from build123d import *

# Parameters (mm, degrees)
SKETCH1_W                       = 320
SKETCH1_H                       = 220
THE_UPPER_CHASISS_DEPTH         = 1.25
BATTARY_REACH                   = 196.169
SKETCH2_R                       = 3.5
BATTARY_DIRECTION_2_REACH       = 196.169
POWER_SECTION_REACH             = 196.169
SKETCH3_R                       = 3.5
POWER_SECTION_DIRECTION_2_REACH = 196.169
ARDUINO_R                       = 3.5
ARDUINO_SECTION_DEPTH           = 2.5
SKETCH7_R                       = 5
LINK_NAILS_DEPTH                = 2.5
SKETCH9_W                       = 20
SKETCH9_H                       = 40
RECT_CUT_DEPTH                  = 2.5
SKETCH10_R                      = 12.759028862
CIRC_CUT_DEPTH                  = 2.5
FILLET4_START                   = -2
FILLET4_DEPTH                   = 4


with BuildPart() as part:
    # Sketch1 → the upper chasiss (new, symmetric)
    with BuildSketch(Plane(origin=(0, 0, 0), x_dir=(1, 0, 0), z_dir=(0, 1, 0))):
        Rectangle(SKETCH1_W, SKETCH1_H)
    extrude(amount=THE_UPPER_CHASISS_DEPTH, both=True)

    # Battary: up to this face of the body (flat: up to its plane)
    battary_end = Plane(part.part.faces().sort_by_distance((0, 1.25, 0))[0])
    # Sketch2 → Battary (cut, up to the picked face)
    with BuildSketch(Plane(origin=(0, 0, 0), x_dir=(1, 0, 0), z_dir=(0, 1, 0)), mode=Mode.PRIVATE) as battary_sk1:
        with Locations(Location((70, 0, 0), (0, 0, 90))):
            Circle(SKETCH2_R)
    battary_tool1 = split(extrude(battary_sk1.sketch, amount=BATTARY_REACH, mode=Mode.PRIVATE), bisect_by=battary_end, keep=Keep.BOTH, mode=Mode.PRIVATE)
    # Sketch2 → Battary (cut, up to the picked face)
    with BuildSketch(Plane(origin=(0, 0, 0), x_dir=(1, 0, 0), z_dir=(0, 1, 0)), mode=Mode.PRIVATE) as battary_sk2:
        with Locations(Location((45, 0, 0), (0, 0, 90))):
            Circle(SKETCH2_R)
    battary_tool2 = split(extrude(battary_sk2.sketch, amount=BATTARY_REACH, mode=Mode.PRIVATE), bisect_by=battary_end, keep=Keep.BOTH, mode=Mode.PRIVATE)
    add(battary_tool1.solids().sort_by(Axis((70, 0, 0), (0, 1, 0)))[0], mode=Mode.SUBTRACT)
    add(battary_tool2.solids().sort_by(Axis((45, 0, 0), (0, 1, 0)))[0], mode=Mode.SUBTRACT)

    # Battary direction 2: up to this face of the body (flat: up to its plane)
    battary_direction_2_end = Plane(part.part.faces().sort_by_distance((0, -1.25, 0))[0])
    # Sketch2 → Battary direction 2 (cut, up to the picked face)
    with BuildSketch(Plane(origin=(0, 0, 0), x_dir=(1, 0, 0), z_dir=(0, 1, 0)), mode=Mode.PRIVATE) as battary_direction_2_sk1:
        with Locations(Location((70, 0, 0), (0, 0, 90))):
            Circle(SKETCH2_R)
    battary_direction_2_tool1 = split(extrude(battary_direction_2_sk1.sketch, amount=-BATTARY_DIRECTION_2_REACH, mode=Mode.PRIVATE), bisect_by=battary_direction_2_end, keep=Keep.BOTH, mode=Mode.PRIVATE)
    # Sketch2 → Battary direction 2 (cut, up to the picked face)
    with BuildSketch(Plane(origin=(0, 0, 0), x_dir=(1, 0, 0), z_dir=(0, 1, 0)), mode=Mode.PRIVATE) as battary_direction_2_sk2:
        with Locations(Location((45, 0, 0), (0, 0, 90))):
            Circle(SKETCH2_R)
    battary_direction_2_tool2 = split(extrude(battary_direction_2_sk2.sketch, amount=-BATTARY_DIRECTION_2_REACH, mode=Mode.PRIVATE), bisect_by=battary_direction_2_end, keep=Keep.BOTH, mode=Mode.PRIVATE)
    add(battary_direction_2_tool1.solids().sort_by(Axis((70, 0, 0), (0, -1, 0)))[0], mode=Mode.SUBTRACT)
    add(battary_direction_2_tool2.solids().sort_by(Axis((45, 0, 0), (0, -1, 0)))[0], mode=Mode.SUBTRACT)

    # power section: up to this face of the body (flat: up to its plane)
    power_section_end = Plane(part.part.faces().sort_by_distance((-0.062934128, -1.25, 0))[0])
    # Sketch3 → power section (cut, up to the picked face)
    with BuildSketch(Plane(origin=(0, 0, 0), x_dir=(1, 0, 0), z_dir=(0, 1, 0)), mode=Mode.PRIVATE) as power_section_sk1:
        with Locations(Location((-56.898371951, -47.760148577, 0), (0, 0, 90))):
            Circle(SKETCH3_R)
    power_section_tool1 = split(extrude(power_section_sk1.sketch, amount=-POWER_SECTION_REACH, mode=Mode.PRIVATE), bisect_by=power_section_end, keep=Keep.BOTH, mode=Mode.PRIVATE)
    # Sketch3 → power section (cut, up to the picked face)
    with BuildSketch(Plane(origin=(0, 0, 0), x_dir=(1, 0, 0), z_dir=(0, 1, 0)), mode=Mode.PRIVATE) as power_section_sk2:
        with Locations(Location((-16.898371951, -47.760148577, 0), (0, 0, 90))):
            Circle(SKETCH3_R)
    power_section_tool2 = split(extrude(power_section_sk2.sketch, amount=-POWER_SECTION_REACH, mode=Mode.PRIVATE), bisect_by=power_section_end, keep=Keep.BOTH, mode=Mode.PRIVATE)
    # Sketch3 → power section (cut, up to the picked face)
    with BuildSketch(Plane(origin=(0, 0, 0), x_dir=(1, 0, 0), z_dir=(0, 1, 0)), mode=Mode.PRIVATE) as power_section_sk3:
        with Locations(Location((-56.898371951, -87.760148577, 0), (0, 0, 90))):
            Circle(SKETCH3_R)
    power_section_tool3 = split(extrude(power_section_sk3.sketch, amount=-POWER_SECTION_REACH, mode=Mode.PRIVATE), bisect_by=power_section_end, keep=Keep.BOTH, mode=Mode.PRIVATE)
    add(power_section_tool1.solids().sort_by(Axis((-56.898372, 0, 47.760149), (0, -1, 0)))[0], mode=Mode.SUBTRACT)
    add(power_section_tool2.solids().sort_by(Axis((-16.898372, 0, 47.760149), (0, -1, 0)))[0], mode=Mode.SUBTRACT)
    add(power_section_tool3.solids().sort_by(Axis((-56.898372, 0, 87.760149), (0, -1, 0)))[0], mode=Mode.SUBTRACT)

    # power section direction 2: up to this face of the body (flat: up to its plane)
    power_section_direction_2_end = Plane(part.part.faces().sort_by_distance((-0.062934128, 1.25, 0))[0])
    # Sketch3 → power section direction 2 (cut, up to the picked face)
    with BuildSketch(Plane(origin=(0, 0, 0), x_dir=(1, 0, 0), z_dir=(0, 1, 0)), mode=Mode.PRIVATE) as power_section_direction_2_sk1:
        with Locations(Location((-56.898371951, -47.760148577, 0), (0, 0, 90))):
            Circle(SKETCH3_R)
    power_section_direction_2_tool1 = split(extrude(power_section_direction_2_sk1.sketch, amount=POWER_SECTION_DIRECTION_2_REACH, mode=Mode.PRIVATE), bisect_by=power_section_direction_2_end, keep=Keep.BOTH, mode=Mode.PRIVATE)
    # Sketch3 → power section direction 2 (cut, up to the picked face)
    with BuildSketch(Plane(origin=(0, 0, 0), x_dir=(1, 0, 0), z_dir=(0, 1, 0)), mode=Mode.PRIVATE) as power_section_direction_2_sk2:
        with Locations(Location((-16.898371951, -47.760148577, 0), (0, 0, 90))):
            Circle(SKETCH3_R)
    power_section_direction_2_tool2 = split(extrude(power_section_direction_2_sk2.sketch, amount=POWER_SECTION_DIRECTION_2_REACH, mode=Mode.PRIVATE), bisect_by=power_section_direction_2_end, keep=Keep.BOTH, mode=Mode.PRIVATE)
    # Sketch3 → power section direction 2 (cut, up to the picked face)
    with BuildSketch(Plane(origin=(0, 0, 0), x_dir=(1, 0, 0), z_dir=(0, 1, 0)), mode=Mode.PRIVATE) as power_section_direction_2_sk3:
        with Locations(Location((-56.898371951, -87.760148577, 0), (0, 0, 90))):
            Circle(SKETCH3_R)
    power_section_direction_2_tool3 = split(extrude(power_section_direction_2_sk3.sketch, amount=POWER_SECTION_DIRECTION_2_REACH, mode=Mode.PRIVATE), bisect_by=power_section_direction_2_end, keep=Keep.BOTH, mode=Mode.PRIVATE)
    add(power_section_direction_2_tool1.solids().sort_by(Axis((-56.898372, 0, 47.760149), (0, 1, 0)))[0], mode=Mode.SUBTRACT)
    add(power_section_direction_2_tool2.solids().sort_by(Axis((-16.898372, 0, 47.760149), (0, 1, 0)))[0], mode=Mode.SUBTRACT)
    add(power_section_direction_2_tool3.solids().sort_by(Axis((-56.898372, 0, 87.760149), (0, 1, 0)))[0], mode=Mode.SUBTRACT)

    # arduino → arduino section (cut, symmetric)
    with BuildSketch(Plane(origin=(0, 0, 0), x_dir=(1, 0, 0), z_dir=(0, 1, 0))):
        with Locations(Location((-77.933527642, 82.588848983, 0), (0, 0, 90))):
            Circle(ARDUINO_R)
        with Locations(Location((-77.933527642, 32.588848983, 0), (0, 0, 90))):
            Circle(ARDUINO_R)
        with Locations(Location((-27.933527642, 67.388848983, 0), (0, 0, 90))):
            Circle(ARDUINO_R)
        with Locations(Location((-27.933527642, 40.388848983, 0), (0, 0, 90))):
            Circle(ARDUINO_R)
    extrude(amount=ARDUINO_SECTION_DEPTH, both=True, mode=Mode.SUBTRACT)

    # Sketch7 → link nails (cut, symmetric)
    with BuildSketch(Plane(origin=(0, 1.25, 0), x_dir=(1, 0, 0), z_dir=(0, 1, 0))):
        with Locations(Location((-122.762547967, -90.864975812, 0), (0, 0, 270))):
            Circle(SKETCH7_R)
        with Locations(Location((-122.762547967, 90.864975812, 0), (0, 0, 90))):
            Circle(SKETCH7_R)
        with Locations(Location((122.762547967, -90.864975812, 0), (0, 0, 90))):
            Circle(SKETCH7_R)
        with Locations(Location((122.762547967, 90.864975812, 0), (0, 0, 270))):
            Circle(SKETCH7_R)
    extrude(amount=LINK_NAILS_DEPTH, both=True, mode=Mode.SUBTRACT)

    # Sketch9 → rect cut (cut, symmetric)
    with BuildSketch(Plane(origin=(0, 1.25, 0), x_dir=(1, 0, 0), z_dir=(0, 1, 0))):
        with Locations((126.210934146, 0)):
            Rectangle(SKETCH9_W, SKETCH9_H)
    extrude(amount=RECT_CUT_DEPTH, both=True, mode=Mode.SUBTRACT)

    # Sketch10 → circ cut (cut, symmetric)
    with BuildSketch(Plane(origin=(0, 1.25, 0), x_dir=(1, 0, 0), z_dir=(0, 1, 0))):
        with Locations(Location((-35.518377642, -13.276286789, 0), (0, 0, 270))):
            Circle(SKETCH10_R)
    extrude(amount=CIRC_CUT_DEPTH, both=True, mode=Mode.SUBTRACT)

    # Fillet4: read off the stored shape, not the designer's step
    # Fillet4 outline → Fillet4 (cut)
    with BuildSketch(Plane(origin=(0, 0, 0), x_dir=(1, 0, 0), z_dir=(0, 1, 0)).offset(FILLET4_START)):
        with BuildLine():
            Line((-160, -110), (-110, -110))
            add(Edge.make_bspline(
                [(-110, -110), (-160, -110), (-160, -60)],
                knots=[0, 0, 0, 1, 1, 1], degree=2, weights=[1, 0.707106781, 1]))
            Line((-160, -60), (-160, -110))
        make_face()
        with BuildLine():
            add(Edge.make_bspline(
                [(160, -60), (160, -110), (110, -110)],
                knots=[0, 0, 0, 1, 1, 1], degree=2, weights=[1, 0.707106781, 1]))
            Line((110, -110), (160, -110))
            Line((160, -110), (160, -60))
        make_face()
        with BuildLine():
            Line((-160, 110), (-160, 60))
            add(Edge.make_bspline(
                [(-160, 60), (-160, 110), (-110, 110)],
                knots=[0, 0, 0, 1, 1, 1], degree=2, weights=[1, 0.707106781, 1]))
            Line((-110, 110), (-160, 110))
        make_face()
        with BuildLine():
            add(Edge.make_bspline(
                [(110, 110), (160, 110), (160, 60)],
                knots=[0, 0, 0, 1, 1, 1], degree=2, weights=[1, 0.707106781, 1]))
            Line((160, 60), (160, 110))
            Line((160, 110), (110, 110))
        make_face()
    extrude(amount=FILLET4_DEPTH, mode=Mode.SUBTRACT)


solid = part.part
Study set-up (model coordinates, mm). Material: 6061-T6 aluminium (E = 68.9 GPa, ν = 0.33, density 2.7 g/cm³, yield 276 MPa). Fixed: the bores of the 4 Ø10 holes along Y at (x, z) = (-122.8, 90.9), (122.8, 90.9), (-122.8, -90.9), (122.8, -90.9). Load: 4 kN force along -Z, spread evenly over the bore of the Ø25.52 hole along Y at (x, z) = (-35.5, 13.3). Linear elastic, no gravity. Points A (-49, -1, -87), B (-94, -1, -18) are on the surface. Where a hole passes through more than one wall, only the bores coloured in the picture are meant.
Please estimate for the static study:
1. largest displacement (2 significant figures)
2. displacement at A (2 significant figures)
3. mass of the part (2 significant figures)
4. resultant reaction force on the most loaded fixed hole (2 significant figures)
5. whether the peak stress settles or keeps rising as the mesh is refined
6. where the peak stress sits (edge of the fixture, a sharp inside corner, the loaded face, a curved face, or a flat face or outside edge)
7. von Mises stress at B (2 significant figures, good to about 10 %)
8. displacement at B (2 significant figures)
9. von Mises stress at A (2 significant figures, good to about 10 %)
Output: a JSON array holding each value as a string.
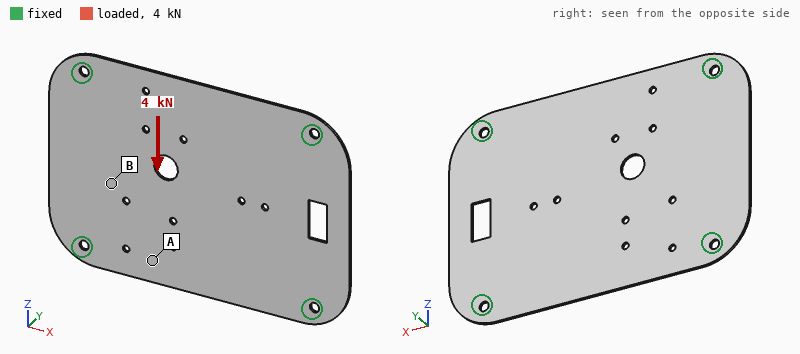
["30 µm", "17 µm", "450 g", "1.5 kN", "keeps rising", "edge of the fixture", "8.2 MPa", "12 µm", "3.8 MPa"]
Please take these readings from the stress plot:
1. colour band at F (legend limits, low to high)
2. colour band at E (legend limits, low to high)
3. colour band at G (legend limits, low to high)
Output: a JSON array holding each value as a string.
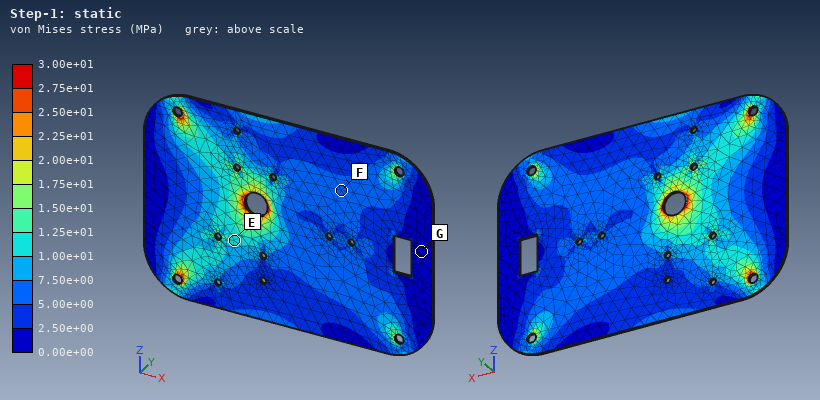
["5.00e+00 to 7.50e+00 MPa", "1.00e+01 to 1.25e+01 MPa", "0.00e+00 to 2.50e+00 MPa"]
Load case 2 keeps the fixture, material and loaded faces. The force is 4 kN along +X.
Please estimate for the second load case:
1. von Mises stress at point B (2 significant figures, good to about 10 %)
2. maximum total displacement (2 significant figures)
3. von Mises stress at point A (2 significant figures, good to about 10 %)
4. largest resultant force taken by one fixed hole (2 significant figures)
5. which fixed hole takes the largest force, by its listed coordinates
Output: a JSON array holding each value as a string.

["5.7 MPa", "23 µm", "2.4 MPa", "1.3 kN", "(-122.8, 90.9)"]
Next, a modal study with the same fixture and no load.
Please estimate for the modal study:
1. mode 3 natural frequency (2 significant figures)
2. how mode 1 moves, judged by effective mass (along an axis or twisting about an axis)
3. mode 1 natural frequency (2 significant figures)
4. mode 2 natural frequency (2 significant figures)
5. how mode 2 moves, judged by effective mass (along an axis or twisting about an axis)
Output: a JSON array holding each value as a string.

["370 Hz", "along Y", "180 Hz", "270 Hz", "twisting about X"]
